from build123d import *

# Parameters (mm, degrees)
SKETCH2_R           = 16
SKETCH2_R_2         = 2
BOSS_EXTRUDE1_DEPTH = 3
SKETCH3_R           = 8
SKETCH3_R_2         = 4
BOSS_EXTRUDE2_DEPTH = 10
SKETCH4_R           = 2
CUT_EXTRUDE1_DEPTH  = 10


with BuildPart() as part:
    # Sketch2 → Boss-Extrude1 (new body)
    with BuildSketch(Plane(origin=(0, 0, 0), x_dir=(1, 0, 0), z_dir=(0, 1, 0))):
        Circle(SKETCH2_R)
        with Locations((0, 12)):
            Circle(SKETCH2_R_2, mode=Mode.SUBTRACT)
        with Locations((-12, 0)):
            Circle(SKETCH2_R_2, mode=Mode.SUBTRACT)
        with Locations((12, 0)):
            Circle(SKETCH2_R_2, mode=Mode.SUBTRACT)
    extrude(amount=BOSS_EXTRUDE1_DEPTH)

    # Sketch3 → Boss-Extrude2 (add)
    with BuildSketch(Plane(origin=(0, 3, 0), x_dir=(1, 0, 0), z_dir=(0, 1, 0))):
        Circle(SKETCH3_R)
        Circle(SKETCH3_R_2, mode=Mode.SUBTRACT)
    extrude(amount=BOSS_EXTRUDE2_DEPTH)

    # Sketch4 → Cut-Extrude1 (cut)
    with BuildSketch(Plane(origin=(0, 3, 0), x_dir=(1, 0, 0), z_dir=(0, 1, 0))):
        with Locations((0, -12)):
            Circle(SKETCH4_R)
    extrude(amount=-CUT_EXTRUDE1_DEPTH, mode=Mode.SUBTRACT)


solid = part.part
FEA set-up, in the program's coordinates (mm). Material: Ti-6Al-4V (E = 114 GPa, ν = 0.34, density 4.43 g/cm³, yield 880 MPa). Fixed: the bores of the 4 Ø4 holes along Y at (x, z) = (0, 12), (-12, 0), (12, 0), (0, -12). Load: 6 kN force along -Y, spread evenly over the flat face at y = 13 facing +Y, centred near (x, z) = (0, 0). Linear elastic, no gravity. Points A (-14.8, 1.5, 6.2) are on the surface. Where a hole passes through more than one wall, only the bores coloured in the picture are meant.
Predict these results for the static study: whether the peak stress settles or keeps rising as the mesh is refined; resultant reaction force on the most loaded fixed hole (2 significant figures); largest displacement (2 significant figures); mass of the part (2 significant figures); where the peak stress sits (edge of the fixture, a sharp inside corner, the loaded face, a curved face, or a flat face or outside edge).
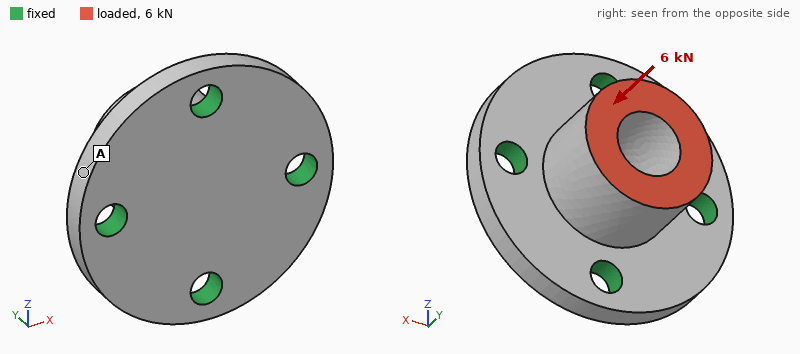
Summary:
keeps rising
1.6 kN
13 µm
17 g
edge of the fixture
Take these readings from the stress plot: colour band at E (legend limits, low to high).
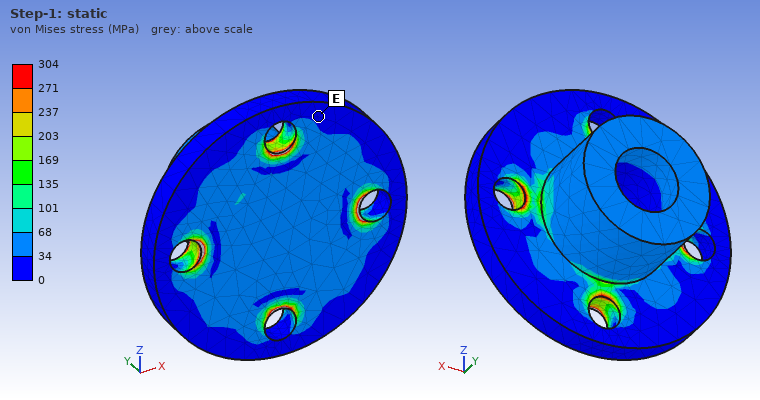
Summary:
0 to 34 MPa
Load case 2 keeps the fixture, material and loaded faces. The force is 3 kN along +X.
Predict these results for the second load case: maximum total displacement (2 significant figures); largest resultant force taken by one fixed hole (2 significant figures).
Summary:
29 µm
2.0 kN
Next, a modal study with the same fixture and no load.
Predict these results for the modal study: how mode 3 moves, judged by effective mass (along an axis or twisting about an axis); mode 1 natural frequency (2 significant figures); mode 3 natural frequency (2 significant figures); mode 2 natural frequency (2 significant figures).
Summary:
along Y
31 kHz
37 kHz
31 kHz
